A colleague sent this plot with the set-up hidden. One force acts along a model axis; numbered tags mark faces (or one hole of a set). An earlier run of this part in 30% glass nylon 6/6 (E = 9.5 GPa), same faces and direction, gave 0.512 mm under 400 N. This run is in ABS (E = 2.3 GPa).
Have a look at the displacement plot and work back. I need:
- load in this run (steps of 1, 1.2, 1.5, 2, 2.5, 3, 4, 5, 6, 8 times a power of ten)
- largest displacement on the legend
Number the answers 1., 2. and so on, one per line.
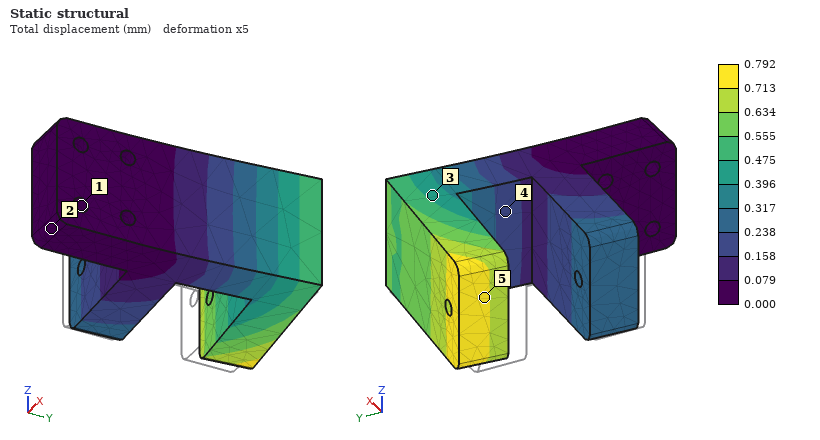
1. 150 N
2. 0.792 mm
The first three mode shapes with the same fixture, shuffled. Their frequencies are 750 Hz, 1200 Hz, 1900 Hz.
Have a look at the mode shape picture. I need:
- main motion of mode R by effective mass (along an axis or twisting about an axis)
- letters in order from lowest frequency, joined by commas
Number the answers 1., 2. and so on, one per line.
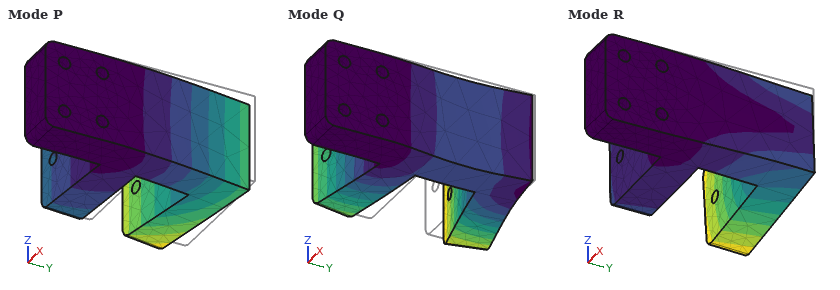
1. along Z
2. P, R, Q
